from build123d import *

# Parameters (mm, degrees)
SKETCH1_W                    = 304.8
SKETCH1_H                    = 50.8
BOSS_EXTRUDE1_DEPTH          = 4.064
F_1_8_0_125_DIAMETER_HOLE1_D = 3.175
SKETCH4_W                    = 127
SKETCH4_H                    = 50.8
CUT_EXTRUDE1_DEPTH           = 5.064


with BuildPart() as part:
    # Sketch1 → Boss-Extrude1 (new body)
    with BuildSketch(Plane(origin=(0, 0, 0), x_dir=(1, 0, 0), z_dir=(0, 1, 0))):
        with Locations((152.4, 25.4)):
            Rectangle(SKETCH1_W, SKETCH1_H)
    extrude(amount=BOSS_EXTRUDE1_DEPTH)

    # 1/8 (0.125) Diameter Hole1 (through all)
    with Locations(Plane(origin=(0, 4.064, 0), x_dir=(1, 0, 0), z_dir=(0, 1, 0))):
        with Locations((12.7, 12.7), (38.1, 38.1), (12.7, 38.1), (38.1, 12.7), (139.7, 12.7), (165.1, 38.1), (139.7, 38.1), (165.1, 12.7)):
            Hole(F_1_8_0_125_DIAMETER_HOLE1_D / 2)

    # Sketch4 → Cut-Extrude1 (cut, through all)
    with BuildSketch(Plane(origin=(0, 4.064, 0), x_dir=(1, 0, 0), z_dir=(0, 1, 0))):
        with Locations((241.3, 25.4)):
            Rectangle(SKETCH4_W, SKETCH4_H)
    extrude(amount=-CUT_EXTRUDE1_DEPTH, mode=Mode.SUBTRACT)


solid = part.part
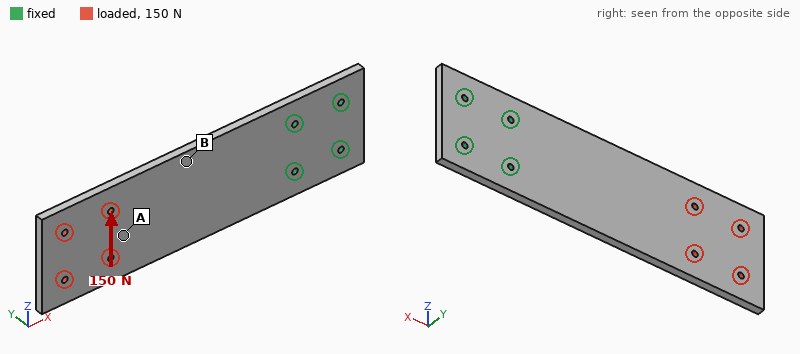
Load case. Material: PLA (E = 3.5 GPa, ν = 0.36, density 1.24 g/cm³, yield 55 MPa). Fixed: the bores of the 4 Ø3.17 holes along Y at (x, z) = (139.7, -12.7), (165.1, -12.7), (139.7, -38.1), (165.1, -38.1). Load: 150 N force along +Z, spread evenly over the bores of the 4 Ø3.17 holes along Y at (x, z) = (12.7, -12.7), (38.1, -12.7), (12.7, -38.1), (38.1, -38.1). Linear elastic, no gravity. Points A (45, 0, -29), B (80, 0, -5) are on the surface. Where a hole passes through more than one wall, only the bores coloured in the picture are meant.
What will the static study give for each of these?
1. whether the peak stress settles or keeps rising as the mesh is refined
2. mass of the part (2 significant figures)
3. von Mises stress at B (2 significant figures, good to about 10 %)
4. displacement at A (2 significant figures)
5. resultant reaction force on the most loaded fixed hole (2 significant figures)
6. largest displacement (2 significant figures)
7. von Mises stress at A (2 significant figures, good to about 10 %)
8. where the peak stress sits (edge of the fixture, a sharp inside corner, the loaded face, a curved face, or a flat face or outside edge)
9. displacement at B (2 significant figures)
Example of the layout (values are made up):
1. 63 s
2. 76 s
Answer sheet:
1. keeps rising
2. 45 g
3. 3.8 MPa
4. 0.52 mm
5. 430 N
6. 0.88 mm
7. 1.8 MPa
8. edge of the fixture
9. 0.29 mm
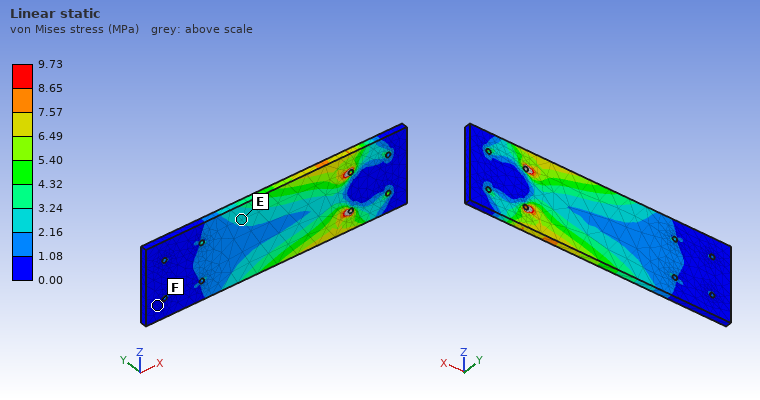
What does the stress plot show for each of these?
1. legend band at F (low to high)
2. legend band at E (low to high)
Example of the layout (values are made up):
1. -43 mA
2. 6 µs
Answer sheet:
1. 0.00 to 1.08 MPa
2. 2.16 to 3.24 MPa
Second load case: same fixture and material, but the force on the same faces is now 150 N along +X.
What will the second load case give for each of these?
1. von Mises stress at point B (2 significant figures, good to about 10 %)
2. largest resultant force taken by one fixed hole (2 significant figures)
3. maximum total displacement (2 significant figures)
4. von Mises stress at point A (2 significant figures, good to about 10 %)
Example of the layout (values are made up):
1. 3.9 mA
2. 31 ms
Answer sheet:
1. 0.73 MPa
2. 60 N
3. 27 µm
4. 0.66 MPa
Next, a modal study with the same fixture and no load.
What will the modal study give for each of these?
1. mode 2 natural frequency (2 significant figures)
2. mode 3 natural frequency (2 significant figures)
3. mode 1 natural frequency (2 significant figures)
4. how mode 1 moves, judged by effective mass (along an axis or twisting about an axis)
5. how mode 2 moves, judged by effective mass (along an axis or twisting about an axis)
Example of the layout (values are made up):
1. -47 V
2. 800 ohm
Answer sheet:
1. 310 Hz
2. 350 Hz
3. 57 Hz
4. along Y
5. twisting about X
